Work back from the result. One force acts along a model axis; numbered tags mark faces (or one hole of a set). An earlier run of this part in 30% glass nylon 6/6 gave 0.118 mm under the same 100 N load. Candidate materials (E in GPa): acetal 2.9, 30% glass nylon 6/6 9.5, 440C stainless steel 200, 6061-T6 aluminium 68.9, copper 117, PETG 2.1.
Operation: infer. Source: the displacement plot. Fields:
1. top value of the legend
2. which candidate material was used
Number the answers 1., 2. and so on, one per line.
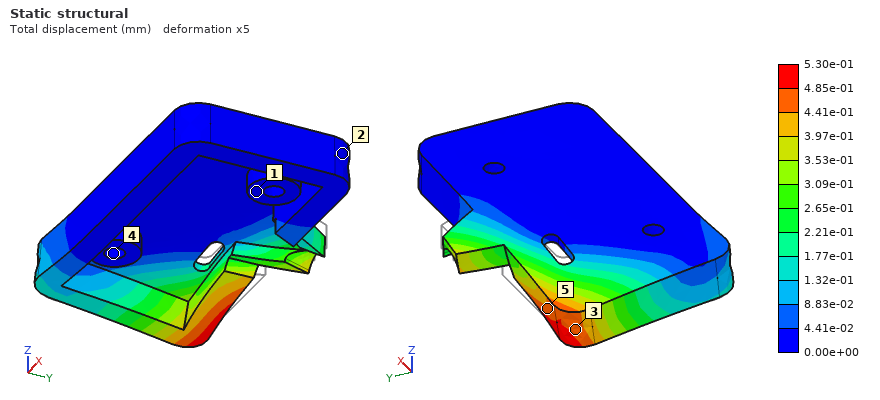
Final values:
1. 5.30e-01 mm
2. PETG
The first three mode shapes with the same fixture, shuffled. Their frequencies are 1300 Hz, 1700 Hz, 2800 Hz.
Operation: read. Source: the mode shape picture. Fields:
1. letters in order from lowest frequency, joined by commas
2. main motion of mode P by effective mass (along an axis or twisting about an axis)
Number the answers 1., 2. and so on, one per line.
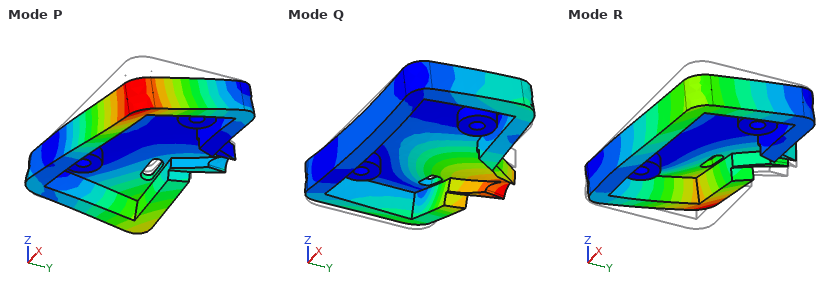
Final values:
1. R, P, Q
2. along Z
